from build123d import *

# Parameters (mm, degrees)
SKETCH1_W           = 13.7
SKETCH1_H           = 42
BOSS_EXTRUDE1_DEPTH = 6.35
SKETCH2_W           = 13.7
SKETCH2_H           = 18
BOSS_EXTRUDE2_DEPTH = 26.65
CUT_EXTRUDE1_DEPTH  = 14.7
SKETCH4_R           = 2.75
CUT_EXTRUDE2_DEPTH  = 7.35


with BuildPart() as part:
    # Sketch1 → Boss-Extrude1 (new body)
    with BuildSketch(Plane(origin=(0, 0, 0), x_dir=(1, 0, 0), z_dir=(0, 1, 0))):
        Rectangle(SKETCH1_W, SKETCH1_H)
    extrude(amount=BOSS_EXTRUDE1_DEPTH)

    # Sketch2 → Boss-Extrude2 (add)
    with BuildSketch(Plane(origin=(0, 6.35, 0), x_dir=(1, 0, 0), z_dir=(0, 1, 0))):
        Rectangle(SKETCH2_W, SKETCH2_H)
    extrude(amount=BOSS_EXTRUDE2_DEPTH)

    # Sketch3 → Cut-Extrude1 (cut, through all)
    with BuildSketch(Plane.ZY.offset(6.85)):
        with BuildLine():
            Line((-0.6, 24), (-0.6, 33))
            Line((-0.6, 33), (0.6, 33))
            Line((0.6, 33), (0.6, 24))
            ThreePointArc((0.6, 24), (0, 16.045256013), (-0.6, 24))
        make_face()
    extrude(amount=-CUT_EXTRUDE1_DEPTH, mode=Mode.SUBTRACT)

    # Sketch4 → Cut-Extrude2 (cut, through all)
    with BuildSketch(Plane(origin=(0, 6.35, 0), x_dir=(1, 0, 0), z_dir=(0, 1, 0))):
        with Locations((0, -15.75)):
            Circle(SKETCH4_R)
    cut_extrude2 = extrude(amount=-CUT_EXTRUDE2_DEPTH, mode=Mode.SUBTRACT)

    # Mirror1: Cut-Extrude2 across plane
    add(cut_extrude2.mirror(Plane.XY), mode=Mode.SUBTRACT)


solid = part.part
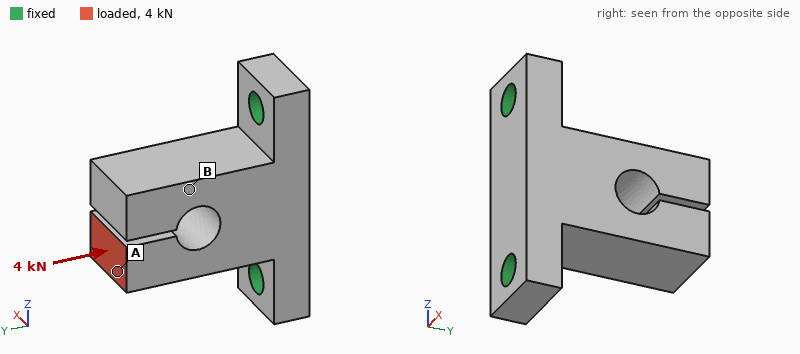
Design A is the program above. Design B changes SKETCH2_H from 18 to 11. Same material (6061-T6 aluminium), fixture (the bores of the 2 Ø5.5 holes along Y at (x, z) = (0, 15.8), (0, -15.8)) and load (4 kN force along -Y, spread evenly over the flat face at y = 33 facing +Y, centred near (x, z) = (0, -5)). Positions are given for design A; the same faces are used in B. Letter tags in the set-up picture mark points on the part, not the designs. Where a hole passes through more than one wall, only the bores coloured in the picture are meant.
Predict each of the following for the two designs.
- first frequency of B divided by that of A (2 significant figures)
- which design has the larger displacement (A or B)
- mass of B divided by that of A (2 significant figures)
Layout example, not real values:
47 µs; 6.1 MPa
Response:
0.62; B; 0.72
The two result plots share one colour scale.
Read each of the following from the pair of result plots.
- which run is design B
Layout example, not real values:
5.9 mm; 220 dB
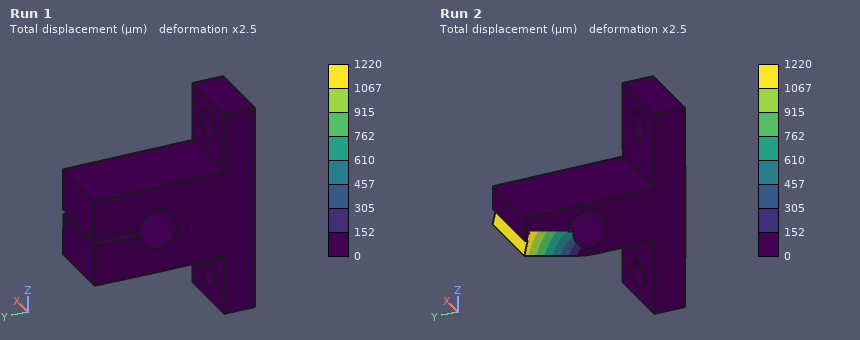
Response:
Run 2
